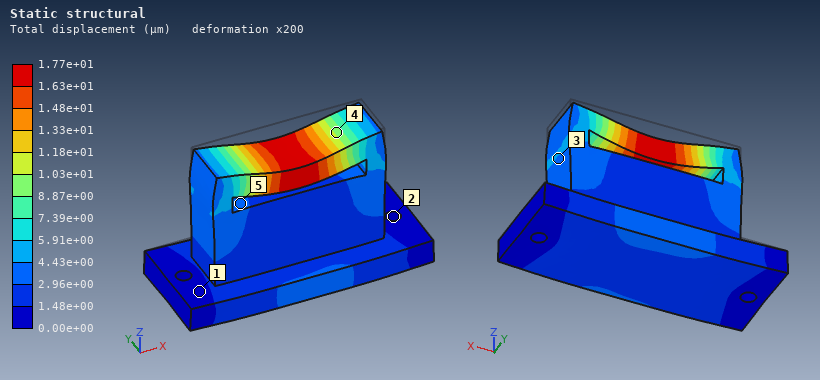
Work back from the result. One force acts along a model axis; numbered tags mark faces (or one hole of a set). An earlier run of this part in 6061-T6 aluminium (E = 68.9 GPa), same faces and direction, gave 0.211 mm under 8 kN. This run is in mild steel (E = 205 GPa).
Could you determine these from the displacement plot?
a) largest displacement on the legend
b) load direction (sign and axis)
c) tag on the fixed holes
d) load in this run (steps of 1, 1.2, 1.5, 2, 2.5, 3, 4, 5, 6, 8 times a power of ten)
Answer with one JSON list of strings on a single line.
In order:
["1.77e+01 µm", "-Z", "2", "2 kN"]
